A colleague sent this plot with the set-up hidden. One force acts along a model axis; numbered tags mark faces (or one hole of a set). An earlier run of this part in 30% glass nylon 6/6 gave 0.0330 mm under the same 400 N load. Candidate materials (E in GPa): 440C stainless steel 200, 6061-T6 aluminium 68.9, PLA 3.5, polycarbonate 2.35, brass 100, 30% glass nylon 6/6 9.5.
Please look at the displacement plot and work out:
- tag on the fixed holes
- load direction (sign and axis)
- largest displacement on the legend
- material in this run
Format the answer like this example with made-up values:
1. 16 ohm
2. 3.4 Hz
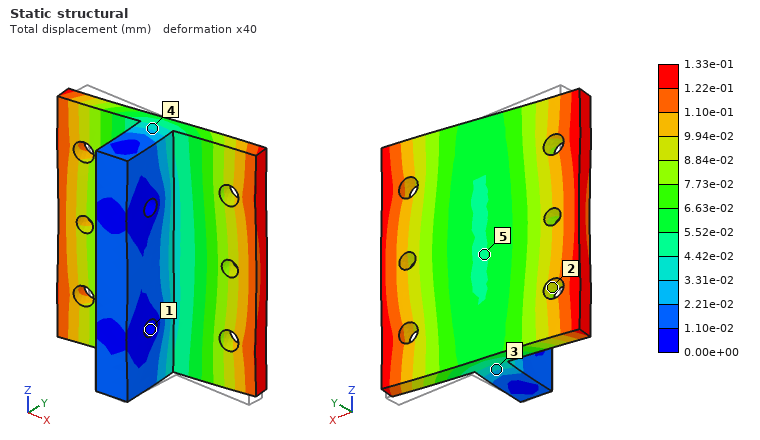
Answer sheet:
1. 1
2. -X
3. 1.33e-01 mm
4. polycarbonate
